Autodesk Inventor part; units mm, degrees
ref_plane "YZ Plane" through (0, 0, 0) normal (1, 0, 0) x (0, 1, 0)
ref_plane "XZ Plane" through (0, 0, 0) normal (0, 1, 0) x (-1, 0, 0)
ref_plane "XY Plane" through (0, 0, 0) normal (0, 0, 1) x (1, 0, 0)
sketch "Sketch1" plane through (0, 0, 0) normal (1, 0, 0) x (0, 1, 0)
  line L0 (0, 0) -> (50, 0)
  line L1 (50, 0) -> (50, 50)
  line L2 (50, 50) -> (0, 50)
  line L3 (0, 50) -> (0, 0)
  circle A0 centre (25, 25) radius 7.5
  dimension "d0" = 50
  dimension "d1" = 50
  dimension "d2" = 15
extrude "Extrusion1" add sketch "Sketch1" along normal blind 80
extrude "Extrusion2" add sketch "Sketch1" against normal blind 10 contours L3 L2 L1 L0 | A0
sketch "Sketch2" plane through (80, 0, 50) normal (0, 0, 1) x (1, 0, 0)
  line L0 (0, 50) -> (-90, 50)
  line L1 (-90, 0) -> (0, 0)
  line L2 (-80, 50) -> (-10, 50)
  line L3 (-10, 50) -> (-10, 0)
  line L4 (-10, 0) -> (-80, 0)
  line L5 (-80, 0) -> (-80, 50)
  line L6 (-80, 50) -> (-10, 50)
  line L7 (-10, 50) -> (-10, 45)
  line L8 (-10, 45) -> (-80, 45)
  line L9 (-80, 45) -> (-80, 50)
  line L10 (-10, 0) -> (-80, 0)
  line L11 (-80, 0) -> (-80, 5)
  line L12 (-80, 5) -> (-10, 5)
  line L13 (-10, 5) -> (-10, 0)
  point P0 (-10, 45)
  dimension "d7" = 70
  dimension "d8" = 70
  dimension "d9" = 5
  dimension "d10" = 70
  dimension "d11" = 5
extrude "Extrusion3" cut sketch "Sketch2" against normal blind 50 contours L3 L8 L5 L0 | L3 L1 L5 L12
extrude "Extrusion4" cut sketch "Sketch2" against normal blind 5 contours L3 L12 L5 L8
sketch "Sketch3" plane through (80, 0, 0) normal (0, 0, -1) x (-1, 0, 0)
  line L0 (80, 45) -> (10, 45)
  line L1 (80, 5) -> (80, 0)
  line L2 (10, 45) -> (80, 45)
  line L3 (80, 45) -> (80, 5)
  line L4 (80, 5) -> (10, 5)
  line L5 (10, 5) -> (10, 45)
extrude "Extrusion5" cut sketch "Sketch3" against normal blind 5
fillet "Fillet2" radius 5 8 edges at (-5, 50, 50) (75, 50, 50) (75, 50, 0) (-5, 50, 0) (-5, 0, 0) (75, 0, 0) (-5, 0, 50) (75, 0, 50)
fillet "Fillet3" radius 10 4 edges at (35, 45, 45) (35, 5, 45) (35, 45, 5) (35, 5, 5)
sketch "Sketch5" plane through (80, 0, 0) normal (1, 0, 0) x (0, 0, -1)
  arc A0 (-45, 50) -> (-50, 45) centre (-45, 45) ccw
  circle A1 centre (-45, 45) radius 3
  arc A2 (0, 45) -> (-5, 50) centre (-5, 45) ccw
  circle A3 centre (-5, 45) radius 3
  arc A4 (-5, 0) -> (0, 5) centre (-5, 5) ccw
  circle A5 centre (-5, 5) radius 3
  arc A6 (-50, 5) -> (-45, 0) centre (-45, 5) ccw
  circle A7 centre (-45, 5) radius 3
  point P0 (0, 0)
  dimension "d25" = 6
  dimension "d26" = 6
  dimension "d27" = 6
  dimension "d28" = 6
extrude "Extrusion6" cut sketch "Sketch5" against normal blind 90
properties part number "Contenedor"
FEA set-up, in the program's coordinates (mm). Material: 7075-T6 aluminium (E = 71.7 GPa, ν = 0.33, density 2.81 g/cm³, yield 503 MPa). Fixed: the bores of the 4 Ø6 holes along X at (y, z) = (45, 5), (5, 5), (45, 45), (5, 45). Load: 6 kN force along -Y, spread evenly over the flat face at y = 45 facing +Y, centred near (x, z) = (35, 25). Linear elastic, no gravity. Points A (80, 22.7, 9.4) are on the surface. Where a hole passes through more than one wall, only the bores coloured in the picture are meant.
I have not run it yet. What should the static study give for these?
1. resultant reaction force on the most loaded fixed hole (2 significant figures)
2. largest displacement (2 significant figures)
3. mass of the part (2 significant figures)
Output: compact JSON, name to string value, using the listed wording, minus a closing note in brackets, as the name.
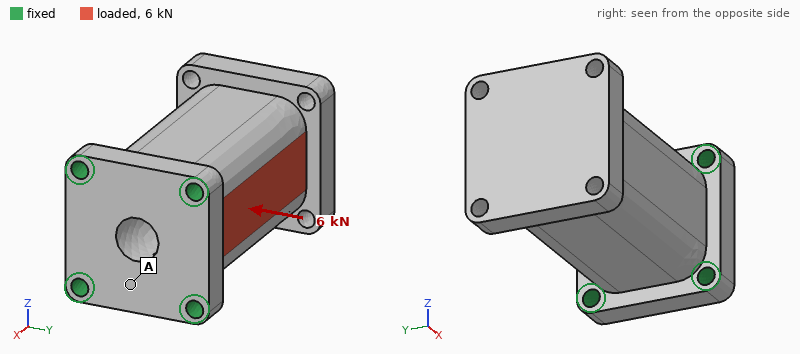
{"resultant reaction force on the most loaded fixed hole": "3.7 kN", "largest displacement": "68 µm", "mass of the part": "390 g"}
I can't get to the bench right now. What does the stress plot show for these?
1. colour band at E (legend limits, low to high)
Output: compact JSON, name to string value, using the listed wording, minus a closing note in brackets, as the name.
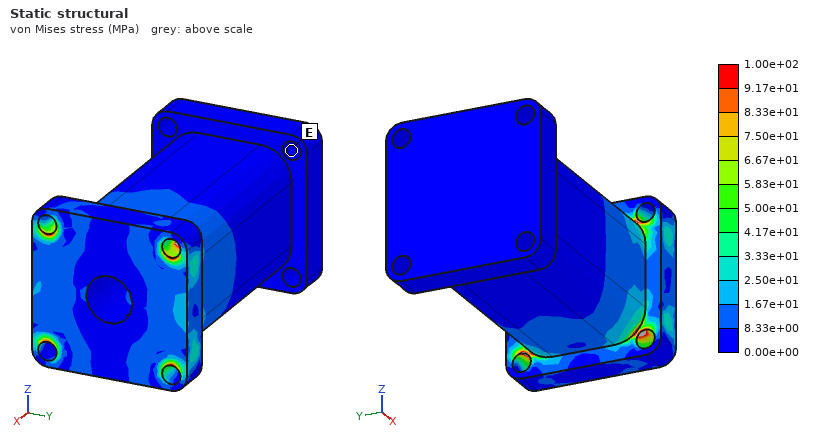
{"colour band at E": "0.00e+00 to 8.33e+00 MPa"}
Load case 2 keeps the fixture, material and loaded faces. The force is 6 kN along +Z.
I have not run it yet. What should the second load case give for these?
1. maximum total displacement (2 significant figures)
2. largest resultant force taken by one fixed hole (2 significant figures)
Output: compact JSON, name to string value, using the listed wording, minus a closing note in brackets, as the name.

{"maximum total displacement": "79 µm", "largest resultant force taken by one fixed hole": "4.0 kN"}
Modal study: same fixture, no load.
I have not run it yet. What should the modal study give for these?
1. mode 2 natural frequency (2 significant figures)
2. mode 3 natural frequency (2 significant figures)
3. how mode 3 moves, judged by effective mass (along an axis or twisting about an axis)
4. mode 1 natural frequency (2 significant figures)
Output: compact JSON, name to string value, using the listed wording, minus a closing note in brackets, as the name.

{"mode 2 natural frequency": "2700 Hz", "mode 3 natural frequency": "7400 Hz", "how mode 3 moves, judged by effective mass": "twisting about X", "mode 1 natural frequency": "2700 Hz"}
